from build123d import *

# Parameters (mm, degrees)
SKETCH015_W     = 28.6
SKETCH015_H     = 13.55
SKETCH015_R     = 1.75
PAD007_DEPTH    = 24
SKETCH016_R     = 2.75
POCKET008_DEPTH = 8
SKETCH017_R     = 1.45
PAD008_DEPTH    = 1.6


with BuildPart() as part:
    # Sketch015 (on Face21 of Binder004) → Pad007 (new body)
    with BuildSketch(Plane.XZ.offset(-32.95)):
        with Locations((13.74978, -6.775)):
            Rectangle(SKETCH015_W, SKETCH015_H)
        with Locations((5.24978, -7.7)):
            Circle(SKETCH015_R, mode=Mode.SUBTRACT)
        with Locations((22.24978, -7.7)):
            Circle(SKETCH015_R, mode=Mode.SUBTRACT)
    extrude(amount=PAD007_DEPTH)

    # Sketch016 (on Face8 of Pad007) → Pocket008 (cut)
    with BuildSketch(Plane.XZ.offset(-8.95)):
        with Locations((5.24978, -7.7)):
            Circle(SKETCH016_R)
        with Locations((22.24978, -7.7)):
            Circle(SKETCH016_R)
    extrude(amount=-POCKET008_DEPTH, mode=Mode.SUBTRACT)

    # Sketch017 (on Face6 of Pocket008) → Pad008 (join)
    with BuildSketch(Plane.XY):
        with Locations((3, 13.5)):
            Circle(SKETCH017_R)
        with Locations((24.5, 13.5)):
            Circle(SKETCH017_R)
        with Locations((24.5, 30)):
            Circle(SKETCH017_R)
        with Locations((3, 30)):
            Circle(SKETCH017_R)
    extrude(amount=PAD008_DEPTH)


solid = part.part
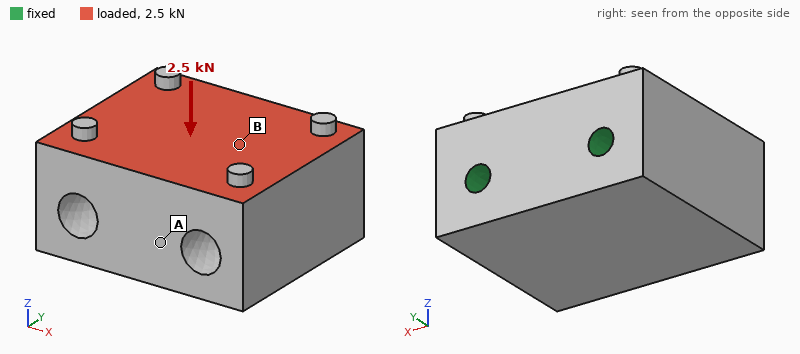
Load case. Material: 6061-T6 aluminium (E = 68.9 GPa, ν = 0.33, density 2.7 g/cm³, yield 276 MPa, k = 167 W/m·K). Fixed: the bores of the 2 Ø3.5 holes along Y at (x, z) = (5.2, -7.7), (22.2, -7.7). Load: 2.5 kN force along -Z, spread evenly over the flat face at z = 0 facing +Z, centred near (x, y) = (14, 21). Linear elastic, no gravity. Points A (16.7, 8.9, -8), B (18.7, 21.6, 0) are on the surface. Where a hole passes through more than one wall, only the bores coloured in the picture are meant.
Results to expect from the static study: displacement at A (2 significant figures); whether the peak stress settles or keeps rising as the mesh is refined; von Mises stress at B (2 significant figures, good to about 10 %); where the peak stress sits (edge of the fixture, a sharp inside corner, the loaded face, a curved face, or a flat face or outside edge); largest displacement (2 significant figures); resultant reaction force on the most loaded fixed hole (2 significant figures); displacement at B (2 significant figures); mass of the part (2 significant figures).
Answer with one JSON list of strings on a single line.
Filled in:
["3.0 µm", "keeps rising", "8.2 MPa", "edge of the fixture", "3.8 µm", "1.3 kN", "1.1 µm", "23 g"]
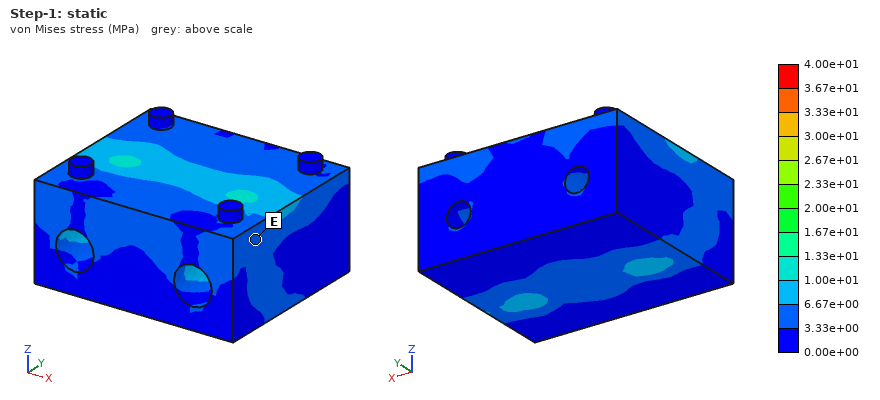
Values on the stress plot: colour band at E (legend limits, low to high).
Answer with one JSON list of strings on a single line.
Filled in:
["3.33e+00 to 6.67e+00 MPa"]
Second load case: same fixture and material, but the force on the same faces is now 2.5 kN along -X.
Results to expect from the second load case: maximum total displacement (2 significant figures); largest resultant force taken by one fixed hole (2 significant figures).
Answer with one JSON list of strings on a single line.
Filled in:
["4.3 µm", "1.6 kN"]
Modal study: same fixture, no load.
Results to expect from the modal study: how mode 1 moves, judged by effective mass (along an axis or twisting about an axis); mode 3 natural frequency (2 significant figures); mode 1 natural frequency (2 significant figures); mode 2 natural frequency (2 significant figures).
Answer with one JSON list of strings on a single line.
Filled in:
["along Z", "48 kHz", "34 kHz", "47 kHz"]
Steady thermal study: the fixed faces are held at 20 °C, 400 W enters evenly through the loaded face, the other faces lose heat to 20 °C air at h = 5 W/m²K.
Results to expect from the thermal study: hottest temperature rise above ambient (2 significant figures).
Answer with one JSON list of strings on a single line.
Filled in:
["50 K"]
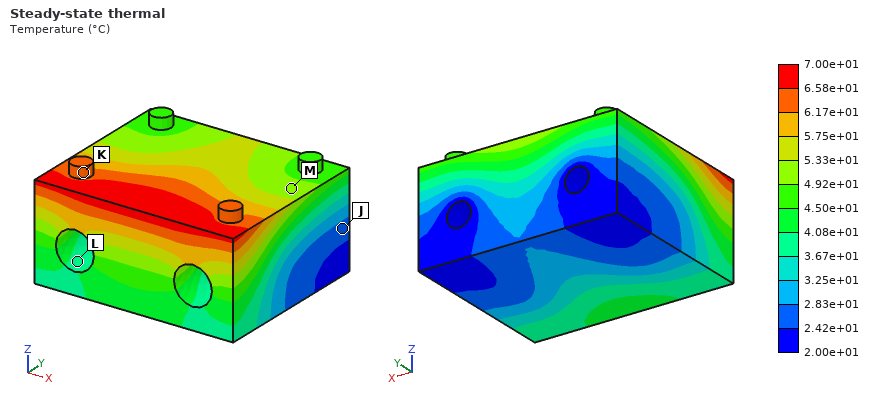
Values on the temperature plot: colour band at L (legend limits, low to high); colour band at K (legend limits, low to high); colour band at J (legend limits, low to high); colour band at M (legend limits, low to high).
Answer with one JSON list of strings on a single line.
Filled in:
["3.67e+01 to 4.08e+01 °C", "6.17e+01 to 6.58e+01 °C", "2.42e+01 to 2.83e+01 °C", "4.92e+01 to 5.33e+01 °C"]
